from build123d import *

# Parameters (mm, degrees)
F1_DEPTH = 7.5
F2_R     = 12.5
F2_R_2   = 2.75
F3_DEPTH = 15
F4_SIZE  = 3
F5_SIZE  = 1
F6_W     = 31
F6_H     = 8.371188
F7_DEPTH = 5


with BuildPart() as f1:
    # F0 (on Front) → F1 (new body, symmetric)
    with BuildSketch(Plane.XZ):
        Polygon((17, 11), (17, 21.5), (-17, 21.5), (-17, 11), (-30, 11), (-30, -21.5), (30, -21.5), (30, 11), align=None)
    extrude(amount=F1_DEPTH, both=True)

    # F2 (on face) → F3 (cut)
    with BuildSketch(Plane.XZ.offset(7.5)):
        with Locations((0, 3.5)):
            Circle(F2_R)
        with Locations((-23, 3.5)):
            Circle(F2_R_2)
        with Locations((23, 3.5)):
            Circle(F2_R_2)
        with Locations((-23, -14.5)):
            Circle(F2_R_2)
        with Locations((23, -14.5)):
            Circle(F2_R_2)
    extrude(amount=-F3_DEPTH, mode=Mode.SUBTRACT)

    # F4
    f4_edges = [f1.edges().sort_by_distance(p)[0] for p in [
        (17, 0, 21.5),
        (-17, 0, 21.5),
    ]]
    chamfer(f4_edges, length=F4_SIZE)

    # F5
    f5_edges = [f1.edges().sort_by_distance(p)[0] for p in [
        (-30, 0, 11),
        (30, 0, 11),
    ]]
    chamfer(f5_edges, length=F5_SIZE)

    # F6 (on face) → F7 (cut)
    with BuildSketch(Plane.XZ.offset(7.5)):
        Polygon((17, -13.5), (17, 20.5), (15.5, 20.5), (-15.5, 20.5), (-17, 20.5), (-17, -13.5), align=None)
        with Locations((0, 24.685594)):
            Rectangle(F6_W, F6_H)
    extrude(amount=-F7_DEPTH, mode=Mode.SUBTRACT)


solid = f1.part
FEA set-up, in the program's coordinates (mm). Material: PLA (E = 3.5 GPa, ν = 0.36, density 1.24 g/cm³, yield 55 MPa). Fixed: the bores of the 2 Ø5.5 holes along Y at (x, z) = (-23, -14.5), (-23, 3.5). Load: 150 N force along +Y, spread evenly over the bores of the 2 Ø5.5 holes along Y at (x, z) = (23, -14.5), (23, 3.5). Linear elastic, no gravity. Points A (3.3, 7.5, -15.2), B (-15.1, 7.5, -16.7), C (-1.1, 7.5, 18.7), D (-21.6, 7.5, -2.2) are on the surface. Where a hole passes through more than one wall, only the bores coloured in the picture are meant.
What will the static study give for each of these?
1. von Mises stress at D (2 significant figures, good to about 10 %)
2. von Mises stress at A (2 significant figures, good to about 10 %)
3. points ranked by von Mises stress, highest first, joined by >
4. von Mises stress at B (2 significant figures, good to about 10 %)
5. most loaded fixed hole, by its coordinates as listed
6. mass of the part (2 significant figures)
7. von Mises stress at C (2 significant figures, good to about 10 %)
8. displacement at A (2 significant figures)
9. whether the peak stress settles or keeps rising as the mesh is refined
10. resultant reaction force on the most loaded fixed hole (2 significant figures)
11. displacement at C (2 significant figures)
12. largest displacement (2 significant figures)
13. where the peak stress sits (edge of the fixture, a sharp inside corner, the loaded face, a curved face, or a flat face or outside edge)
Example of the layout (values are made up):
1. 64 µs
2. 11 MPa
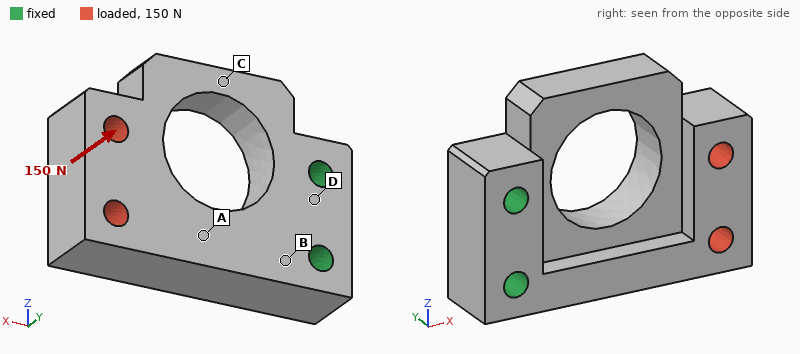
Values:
1. 2.9 MPa
2. 6.3 MPa
3. B > A > C > D
4. 10 MPa
5. (-23, -14.5)
6. 28 g
7. 4.8 MPa
8. 0.16 mm
9. keeps rising
10. 87 N
11. 0.14 mm
12. 0.55 mm
13. edge of the fixture
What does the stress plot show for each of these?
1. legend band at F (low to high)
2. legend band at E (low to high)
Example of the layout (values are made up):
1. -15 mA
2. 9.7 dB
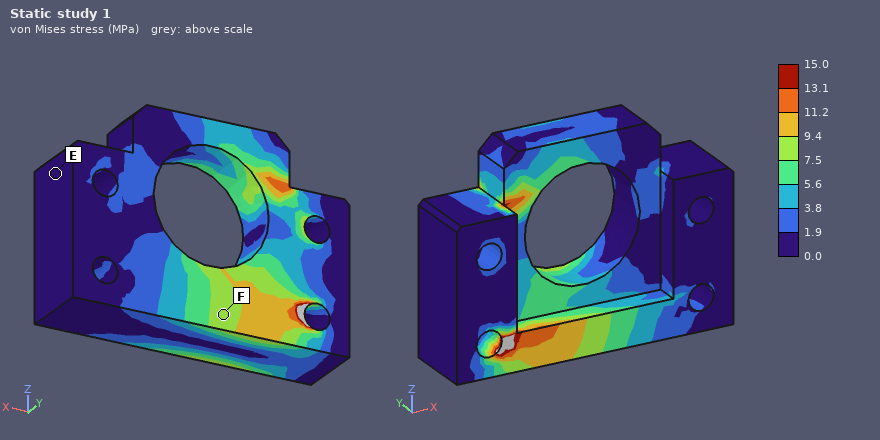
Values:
1. 7.5 to 9.4 MPa
2. 0.0 to 1.9 MPa
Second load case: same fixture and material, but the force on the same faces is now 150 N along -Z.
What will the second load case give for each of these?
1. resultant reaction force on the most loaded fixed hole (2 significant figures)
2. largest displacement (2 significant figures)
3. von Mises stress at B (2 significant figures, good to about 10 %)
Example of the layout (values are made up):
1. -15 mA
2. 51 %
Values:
1. 310 N
2. 0.21 mm
3. 3.7 MPa
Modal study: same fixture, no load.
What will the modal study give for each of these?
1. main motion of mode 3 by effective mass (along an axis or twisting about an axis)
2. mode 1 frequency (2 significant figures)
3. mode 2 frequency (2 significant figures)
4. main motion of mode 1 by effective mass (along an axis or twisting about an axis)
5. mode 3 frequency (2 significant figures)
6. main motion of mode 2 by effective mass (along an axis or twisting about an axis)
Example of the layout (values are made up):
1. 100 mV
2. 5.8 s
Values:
1. twisting about X
2. 950 Hz
3. 1400 Hz
4. along Y
5. 2200 Hz
6. along Z
